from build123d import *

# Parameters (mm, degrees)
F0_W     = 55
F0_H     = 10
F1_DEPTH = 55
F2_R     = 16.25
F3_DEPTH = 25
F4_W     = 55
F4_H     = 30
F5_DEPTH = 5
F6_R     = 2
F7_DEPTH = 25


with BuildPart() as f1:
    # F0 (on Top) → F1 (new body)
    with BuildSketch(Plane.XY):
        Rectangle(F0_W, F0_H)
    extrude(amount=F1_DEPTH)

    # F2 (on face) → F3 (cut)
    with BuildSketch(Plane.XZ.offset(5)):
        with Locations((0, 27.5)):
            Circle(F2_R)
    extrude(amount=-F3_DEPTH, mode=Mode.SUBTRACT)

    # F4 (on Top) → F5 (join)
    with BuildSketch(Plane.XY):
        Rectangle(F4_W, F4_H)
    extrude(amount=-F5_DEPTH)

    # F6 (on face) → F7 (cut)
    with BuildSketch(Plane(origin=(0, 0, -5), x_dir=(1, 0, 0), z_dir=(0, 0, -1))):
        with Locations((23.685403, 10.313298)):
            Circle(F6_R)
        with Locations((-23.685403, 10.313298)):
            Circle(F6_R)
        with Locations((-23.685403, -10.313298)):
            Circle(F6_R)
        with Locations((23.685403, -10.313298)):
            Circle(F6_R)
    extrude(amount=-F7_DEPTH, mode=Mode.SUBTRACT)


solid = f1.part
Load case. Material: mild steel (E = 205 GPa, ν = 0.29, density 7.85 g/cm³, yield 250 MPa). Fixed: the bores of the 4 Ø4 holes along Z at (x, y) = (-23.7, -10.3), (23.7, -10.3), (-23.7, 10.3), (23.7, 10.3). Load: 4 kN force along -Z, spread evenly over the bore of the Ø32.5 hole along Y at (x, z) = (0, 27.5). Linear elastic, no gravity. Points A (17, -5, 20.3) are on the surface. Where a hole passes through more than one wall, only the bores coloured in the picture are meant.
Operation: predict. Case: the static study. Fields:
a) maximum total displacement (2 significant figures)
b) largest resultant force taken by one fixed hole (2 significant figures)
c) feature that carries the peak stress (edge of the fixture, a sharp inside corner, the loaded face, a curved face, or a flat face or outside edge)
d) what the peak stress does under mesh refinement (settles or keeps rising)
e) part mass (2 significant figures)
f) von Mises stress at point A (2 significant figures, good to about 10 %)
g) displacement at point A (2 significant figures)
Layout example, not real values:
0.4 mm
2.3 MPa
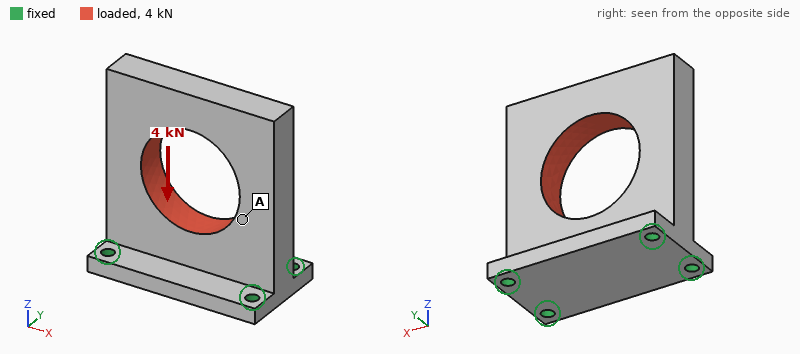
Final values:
6.3 µm
1.0 kN
edge of the fixture
keeps rising
240 g
13 MPa
3.6 µm
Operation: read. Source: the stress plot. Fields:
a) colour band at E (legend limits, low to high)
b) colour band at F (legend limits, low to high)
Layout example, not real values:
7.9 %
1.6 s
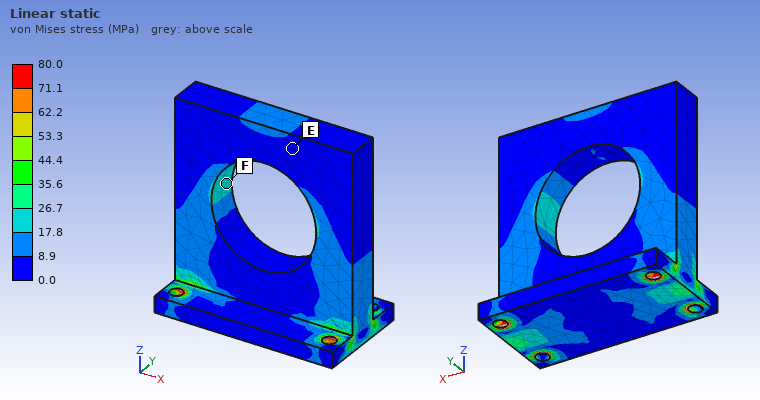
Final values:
0.0 to 8.9 MPa
17.8 to 26.7 MPa
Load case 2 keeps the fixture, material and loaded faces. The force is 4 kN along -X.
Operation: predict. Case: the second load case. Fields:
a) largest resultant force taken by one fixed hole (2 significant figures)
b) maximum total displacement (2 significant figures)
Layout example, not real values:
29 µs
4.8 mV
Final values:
1.7 kN
28 µm
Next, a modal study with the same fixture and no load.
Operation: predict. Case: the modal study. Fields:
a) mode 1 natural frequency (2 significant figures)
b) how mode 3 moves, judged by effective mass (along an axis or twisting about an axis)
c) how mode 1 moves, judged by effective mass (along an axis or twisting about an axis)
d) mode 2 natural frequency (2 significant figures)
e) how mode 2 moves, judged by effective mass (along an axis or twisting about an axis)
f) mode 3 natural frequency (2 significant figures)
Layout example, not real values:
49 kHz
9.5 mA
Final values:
1900 Hz
along X
along Y
4500 Hz
twisting about Z
5100 Hz
